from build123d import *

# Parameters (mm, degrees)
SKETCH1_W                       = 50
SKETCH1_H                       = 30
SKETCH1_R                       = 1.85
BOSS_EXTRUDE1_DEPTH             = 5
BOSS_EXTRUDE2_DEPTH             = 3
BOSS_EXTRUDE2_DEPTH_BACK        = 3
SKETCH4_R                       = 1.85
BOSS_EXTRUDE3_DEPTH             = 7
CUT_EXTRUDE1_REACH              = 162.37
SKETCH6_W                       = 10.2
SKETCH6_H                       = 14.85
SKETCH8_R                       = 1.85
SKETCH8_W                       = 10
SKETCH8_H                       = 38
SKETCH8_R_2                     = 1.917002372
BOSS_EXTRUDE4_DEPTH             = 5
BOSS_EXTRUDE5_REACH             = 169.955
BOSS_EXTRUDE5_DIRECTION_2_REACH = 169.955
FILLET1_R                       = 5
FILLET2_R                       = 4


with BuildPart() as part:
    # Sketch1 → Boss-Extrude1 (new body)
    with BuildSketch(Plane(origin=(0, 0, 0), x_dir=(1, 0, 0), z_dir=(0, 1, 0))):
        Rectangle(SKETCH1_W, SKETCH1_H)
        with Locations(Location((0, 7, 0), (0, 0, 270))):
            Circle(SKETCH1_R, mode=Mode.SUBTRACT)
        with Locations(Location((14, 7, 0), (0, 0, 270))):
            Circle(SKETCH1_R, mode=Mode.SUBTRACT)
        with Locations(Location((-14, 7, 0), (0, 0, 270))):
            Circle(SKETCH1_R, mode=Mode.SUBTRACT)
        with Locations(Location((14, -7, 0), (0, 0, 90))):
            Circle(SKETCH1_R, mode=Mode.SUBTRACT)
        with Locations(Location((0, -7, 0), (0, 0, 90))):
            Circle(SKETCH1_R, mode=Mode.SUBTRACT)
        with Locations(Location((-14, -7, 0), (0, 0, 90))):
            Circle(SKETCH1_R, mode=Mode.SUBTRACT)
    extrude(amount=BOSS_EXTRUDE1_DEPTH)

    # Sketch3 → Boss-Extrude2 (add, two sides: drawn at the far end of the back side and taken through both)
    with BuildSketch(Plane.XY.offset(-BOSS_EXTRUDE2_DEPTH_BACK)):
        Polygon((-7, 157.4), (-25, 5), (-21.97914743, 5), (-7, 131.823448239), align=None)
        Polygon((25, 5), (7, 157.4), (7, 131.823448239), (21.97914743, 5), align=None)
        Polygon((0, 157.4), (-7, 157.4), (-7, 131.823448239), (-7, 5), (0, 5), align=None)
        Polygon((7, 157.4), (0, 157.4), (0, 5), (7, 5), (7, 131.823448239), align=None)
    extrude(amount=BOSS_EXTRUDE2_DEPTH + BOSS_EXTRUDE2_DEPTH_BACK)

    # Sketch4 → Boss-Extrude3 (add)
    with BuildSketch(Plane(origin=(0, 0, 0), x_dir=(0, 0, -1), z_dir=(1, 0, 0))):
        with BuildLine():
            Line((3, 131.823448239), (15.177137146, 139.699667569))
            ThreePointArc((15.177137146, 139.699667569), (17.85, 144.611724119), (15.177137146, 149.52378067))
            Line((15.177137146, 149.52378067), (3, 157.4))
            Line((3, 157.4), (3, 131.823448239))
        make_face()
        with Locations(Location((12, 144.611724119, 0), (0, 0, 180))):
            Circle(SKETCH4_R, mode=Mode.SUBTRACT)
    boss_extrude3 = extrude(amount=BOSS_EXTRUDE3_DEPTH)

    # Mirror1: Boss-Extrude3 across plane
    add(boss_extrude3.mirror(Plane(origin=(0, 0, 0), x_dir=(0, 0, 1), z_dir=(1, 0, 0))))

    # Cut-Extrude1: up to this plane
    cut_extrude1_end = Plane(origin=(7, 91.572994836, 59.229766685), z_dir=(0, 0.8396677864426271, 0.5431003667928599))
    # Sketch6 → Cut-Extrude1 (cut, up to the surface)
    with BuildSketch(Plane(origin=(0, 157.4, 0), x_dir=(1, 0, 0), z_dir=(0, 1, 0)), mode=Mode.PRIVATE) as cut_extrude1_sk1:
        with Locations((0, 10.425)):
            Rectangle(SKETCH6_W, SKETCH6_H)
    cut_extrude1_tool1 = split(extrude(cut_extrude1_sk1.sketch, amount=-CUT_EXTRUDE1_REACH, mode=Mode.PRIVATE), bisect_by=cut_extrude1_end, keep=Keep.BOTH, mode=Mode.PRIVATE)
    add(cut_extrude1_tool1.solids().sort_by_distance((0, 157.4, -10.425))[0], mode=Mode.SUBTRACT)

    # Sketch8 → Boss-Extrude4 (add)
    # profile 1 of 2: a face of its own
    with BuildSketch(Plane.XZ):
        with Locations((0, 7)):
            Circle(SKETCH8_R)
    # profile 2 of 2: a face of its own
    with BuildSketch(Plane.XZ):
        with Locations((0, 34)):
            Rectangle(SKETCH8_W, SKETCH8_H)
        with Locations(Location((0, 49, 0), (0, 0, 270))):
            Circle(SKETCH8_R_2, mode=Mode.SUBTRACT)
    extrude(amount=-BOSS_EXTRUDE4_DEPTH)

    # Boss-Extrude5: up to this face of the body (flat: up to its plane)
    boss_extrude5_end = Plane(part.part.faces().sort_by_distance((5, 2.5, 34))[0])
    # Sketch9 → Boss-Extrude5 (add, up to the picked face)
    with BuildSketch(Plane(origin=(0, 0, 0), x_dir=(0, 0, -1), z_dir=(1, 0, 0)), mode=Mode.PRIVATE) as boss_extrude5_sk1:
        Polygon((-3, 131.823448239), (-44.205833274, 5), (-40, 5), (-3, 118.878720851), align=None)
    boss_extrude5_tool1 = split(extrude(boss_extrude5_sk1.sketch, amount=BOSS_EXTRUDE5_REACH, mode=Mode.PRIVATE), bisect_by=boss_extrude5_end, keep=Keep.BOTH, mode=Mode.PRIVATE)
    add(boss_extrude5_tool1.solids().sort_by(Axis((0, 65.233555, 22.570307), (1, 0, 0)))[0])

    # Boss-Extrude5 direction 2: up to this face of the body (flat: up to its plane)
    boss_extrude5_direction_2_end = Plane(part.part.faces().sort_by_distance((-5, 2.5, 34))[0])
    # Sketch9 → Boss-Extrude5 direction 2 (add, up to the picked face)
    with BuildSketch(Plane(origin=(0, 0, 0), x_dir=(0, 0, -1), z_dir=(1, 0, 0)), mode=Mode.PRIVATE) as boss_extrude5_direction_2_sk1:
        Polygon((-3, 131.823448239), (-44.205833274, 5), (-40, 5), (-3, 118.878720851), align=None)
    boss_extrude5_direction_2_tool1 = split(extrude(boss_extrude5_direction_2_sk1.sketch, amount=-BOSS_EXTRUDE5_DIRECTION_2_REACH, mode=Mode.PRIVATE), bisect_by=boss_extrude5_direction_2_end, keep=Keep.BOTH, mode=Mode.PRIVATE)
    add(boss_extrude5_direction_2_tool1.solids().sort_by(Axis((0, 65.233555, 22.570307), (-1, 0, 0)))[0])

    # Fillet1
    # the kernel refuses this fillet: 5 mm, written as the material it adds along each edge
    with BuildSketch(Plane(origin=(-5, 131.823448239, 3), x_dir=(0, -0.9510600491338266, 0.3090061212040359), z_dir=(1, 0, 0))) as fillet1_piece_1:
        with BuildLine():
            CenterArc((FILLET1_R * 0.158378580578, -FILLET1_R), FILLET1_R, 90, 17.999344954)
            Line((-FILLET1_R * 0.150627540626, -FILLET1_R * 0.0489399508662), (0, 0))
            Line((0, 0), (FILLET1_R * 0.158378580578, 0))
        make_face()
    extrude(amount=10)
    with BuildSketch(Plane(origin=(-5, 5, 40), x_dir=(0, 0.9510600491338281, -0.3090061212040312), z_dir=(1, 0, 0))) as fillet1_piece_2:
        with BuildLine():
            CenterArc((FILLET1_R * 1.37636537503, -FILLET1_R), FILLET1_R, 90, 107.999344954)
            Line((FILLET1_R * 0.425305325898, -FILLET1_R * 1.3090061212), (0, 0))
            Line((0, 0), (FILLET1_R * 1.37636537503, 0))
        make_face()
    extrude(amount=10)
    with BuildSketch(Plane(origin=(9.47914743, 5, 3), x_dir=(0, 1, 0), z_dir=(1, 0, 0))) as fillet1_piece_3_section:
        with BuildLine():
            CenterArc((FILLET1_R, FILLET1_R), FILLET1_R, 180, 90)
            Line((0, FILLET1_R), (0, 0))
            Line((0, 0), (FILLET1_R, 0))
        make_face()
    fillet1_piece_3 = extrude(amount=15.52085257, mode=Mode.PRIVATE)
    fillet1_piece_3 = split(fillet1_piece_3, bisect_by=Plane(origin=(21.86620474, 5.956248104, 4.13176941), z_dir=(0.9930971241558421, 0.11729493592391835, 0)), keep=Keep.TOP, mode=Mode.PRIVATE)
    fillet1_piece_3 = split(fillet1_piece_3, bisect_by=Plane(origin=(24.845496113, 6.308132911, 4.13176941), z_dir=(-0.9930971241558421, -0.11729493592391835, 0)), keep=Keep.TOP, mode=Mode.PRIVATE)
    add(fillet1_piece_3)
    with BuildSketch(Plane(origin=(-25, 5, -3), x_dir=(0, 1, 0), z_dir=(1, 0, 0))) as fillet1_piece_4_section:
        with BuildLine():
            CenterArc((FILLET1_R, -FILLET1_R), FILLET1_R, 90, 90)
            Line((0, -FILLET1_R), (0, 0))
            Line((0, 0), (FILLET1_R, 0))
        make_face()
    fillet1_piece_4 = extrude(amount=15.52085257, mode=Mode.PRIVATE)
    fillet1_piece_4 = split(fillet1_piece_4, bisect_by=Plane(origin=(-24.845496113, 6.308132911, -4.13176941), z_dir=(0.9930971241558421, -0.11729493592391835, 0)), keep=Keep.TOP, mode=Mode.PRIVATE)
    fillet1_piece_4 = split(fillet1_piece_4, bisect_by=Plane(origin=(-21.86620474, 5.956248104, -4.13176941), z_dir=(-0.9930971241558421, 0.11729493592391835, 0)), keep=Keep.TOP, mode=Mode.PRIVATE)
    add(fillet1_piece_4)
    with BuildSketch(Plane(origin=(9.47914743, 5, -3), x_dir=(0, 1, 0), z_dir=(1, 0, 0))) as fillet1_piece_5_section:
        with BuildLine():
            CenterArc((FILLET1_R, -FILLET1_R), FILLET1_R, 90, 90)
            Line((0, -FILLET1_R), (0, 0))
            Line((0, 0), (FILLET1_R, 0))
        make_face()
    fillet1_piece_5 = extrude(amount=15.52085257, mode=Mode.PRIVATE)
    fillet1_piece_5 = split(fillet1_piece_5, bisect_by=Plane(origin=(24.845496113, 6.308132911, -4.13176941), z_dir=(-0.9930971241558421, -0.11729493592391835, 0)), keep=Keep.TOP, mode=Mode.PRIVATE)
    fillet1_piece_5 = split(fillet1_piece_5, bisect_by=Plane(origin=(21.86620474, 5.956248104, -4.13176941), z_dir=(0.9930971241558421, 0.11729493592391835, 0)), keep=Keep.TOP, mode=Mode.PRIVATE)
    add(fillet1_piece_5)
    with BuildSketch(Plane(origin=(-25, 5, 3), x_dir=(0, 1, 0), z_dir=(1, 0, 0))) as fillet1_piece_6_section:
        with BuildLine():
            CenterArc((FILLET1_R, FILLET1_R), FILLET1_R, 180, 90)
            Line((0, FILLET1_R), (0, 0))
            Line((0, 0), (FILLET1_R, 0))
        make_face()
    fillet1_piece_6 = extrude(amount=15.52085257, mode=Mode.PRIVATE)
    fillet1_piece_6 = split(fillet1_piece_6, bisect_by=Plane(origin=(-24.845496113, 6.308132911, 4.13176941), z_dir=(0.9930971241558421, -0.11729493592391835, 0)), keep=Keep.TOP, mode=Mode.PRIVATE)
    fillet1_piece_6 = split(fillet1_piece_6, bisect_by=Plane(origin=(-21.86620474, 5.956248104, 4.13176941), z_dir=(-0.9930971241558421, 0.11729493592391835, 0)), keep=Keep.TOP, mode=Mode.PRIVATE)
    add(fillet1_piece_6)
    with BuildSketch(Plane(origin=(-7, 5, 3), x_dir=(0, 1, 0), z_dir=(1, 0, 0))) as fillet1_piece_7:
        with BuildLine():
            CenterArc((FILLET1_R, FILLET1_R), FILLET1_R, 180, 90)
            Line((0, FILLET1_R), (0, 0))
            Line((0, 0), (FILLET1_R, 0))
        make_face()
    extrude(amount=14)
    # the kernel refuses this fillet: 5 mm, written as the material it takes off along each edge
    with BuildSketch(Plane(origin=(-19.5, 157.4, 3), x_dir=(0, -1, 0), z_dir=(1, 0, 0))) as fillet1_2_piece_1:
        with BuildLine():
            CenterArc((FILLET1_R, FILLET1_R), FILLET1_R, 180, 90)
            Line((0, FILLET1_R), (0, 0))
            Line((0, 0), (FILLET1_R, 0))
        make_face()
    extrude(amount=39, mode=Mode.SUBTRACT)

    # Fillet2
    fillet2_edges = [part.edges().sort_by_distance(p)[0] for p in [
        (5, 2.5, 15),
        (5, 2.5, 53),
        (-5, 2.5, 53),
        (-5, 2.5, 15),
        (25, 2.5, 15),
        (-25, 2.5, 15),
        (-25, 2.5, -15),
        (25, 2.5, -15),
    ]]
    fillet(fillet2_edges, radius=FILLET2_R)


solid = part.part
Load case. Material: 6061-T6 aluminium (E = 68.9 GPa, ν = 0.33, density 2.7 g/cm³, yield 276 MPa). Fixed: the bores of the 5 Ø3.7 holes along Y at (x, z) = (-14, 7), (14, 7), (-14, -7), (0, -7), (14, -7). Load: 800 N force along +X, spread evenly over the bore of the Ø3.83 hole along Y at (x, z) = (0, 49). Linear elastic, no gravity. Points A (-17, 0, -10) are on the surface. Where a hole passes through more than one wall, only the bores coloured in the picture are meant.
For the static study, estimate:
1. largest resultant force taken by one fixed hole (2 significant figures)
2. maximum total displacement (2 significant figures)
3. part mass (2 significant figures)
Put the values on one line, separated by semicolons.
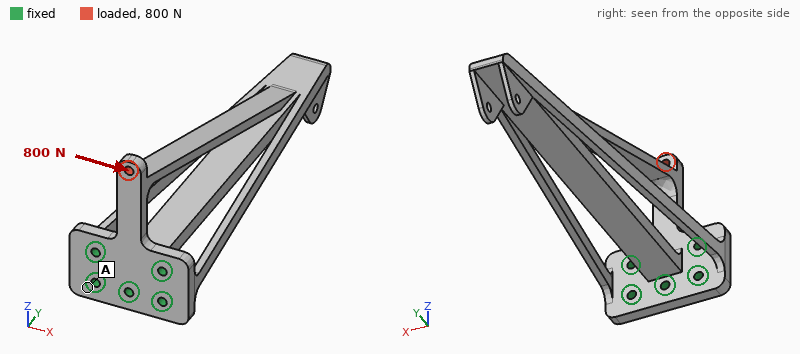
1.1 kN; 0.48 mm; 89 g
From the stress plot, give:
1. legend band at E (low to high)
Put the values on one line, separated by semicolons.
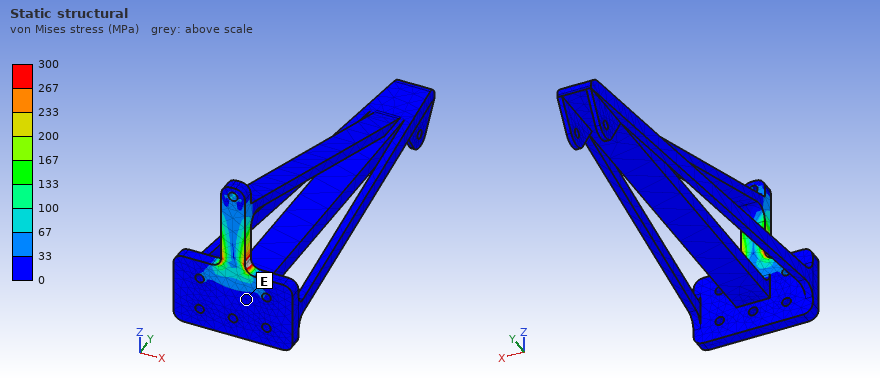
0 to 33 MPa
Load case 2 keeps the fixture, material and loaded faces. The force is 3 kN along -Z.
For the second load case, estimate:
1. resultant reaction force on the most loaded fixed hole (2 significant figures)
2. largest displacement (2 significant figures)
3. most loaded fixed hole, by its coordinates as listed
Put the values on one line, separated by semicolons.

1000 N; 48 µm; (0, -7)
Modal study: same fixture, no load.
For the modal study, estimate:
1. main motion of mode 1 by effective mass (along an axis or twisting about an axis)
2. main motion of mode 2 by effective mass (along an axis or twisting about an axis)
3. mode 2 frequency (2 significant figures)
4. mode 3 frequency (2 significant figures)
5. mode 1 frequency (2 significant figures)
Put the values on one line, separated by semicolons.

along Z; along X; 710 Hz; 920 Hz; 310 Hz
